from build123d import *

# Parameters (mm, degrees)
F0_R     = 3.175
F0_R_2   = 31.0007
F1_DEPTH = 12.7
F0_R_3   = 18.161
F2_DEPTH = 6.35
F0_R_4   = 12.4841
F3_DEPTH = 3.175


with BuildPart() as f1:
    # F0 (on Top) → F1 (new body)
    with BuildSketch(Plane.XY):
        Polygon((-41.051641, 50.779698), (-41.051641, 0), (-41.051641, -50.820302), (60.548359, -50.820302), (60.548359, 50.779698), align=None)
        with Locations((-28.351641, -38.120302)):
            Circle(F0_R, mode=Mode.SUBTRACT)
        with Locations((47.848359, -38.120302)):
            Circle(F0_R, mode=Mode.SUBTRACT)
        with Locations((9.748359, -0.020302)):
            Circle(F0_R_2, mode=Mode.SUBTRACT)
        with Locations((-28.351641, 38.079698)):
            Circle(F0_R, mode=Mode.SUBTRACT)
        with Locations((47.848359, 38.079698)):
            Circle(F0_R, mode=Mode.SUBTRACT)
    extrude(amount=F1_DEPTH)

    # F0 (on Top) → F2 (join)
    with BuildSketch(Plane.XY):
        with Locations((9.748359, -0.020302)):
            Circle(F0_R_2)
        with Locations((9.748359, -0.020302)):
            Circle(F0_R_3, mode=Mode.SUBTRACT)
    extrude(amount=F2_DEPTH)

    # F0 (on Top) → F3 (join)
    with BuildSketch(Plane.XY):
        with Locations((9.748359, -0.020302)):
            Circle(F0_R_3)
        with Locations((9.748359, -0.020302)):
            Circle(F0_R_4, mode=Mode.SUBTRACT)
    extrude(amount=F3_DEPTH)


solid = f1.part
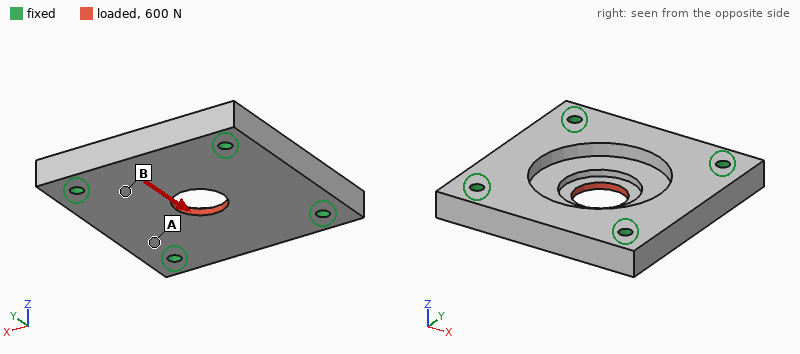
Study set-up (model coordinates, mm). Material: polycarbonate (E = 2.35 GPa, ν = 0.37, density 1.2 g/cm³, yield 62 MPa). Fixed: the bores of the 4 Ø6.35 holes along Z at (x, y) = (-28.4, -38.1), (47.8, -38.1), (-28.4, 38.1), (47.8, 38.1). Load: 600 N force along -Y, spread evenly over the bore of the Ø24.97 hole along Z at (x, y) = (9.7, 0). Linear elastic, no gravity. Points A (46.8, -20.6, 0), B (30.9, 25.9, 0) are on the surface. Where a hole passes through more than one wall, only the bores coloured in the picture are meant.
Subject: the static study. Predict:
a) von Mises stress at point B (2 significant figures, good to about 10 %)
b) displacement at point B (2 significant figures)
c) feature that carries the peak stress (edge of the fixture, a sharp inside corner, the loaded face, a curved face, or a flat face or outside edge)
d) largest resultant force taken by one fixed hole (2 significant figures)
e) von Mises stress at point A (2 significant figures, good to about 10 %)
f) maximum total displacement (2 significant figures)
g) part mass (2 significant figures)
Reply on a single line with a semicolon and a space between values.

1.1 MPa; 10 µm; a sharp inside corner; 160 N; 0.41 MPa; 43 µm; 130 g
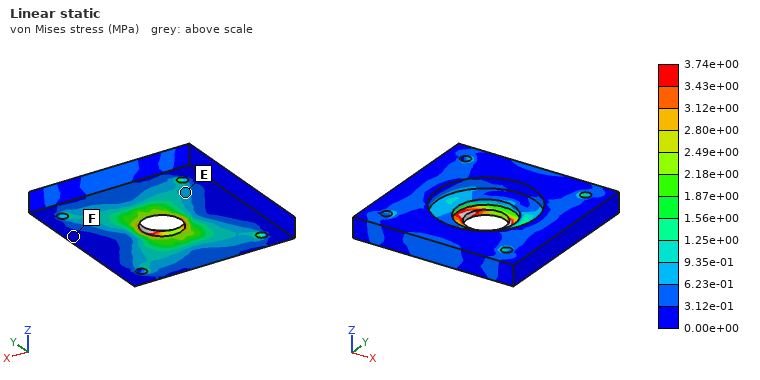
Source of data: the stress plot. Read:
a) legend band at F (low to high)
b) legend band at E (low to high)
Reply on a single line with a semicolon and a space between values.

0.00e+00 to 3.12e-01 MPa; 6.23e-01 to 9.35e-01 MPa
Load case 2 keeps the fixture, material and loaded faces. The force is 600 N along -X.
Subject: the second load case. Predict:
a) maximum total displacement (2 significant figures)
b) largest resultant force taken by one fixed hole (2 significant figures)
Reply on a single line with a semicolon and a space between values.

43 µm; 160 N
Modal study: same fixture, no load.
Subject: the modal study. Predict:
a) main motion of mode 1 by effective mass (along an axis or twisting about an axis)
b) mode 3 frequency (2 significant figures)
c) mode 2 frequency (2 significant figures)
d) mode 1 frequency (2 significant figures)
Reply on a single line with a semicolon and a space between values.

along Z; 2600 Hz; 2600 Hz; 2200 Hz
